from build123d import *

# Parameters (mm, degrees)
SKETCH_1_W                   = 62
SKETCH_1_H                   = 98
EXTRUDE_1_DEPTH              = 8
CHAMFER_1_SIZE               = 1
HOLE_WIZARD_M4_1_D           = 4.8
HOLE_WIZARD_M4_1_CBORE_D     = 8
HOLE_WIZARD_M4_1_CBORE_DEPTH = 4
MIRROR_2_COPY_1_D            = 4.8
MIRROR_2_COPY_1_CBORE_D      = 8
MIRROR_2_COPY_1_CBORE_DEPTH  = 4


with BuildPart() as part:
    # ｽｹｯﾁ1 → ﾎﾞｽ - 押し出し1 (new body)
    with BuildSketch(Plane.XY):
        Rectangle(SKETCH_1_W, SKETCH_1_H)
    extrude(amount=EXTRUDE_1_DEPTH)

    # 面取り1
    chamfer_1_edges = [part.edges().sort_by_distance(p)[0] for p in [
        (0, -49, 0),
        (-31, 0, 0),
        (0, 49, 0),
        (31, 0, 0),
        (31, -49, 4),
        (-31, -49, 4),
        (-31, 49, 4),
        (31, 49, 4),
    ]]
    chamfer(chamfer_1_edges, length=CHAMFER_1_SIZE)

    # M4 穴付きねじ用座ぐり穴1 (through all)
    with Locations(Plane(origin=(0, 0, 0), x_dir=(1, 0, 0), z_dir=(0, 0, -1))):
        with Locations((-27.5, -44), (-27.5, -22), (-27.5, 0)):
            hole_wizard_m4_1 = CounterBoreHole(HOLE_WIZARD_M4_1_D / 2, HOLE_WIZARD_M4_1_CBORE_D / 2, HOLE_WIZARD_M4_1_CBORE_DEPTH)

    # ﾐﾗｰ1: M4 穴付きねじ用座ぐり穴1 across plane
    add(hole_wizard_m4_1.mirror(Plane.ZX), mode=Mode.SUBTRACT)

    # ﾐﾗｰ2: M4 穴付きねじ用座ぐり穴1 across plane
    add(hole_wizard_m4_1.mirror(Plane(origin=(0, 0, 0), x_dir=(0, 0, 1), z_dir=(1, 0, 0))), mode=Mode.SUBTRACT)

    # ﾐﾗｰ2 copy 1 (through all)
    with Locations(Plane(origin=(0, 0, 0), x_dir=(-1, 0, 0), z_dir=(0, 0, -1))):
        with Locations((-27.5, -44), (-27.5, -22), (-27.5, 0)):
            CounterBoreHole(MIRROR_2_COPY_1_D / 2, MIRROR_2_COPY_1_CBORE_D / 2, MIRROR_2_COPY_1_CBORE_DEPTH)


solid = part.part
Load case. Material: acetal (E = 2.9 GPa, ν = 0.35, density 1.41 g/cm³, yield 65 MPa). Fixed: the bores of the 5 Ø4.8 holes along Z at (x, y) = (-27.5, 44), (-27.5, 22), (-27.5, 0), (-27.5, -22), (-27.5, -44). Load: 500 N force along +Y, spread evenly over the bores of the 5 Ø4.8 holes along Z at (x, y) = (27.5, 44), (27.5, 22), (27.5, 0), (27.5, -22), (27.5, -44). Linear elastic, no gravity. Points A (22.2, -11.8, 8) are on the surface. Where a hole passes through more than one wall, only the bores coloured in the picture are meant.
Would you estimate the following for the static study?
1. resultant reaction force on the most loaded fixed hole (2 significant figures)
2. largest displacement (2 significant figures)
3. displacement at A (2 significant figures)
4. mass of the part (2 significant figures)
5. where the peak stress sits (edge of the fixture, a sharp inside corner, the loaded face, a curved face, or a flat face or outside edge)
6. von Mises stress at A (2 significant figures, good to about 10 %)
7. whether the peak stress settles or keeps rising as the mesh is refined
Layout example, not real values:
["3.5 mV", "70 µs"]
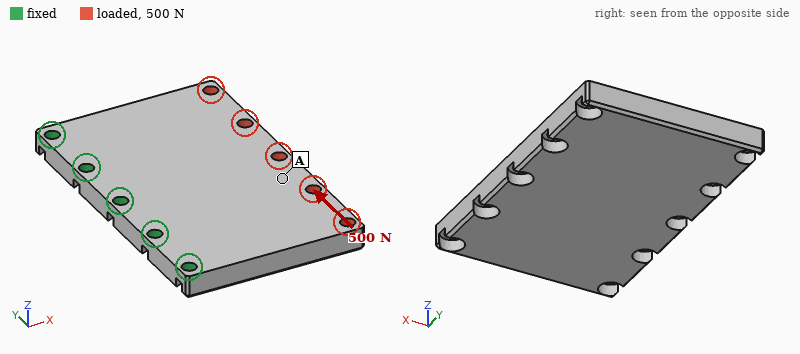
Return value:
["270 N", "0.21 mm", "0.081 mm", "65 g", "edge of the fixture", "2.2 MPa", "keeps rising"]
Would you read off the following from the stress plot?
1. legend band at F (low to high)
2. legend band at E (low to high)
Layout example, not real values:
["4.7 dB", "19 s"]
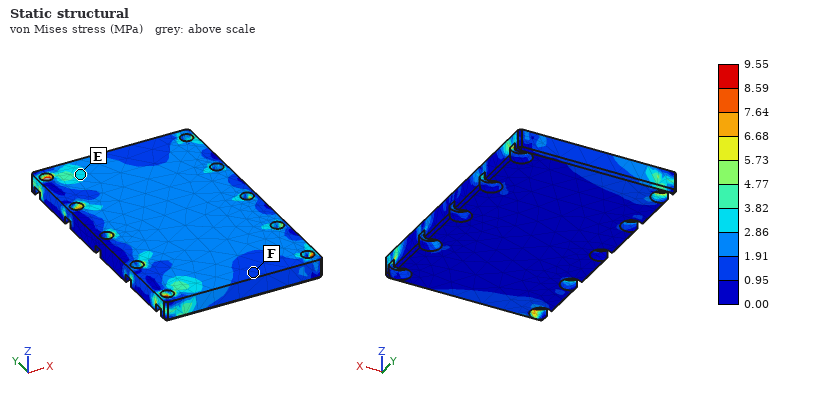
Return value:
["0.95 to 1.91 MPa", "2.86 to 3.82 MPa"]
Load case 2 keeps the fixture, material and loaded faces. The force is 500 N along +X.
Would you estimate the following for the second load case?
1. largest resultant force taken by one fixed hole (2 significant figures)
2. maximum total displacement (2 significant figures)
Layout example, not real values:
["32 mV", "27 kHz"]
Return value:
["100 N", "0.13 mm"]
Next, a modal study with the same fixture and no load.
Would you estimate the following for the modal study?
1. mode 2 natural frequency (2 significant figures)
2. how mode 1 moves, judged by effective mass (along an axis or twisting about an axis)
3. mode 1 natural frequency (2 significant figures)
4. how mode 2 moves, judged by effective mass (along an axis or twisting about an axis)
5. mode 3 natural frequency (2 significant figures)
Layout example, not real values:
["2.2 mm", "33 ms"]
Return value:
["780 Hz", "along Z", "390 Hz", "twisting about X", "1800 Hz"]
